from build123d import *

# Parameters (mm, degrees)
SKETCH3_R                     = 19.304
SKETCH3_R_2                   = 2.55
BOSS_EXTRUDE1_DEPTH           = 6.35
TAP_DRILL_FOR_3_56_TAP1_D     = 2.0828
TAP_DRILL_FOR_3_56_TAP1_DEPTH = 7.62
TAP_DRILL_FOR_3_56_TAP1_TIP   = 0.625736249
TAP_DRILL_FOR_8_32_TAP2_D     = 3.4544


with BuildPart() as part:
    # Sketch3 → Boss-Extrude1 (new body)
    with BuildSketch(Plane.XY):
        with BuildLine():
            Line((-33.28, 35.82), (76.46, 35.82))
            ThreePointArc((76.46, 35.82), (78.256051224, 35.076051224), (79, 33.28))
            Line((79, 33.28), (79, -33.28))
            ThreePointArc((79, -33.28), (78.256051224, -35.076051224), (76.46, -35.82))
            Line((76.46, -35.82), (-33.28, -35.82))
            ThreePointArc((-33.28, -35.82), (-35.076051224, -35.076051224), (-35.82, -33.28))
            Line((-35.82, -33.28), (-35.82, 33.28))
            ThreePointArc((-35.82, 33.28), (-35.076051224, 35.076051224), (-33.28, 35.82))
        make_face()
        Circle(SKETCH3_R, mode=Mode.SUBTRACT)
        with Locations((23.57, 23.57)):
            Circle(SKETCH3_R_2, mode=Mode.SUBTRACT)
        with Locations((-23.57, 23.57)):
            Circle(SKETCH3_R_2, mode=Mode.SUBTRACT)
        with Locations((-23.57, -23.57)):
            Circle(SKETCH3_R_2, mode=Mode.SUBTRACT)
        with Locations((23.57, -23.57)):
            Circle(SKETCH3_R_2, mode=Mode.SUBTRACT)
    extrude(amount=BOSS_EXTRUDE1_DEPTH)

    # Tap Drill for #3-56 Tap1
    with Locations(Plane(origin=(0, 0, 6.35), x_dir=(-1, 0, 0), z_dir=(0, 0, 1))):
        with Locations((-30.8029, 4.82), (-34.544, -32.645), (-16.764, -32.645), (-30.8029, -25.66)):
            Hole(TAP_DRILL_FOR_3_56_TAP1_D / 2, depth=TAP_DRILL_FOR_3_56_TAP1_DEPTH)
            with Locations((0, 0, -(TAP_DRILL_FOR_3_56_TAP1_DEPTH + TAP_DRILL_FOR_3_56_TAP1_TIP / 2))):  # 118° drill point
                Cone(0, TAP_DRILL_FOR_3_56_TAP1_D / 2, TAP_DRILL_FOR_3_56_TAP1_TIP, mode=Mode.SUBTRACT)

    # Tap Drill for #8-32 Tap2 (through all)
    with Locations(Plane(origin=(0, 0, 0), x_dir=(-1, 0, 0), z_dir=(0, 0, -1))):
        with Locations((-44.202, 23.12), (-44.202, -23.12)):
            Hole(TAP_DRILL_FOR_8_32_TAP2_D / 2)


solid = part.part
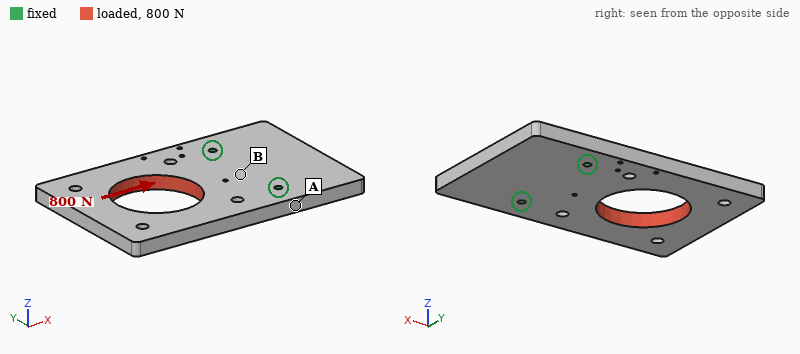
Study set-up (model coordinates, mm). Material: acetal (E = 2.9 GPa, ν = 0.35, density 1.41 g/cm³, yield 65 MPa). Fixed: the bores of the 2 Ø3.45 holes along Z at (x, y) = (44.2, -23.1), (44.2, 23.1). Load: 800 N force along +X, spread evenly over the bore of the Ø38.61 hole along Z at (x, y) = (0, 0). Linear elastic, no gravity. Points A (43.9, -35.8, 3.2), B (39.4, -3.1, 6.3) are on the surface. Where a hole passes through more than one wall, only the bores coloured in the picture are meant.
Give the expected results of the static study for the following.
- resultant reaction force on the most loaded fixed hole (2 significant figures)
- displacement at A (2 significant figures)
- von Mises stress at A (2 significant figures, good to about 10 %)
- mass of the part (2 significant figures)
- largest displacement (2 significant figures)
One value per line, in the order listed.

400 N
15 µm
1.7 MPa
62 g
96 µm
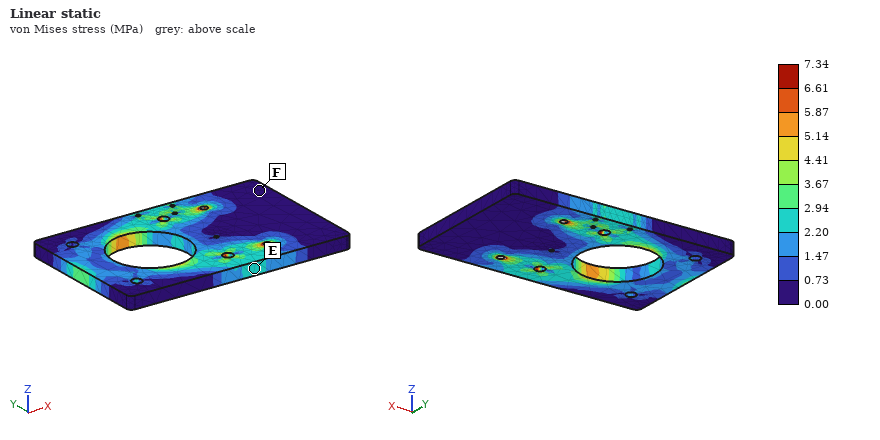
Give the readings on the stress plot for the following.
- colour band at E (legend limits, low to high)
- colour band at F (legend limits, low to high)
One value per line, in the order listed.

2.20 to 2.94 MPa
0.00 to 0.73 MPa
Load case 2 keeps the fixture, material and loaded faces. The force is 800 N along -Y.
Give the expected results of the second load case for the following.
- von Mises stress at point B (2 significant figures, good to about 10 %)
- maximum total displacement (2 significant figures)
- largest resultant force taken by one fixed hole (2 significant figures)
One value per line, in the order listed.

4.7 MPa
0.48 mm
840 N
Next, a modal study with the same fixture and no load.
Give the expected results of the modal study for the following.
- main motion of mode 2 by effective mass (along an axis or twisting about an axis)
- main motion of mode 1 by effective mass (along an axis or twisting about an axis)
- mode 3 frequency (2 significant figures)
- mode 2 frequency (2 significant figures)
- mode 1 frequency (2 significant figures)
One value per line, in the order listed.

twisting about X
along Z
940 Hz
500 Hz
200 Hz
